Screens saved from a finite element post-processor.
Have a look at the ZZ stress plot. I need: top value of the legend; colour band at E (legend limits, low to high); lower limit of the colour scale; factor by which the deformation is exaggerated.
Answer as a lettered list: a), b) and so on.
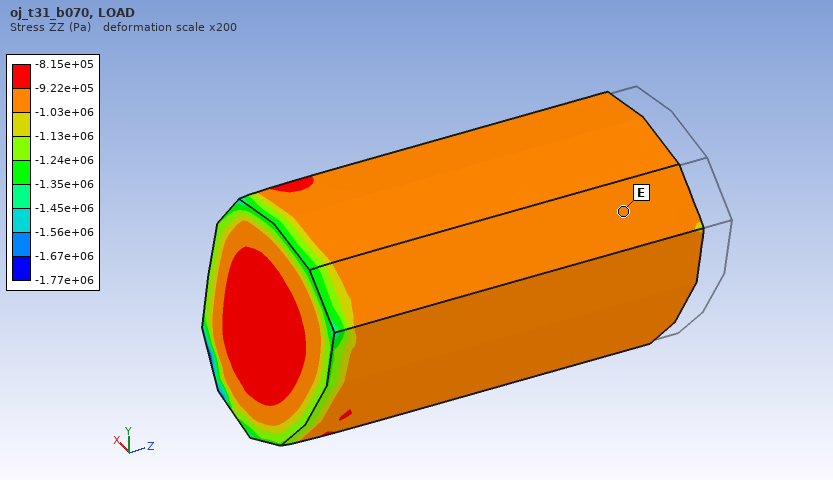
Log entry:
a) -8.15e+05 Pa
b) -1.03e+06 to -9.22e+05 Pa
c) -1.77e+06 Pa
d) 200
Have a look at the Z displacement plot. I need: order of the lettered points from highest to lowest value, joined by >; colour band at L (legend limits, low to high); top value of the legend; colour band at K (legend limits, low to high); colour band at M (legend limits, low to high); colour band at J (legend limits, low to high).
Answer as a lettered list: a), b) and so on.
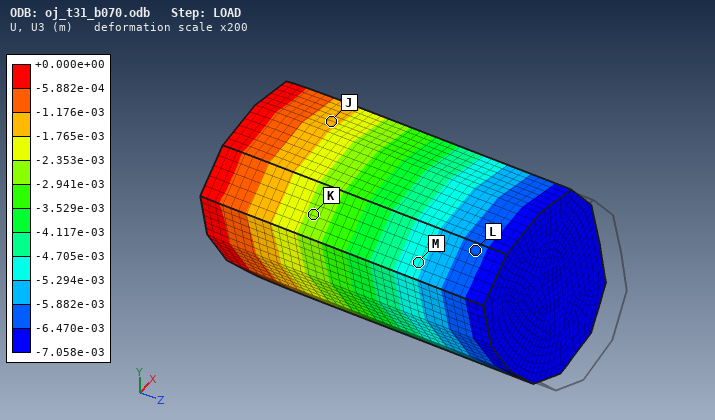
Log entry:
a) J > K > M > L
b) -6.470e-03 to -5.882e-03 m
c) +0.000e+00 m
d) -2.941e-03 to -2.353e-03 m
e) -5.294e-03 to -4.705e-03 m
f) -1.765e-03 to -1.176e-03 m
